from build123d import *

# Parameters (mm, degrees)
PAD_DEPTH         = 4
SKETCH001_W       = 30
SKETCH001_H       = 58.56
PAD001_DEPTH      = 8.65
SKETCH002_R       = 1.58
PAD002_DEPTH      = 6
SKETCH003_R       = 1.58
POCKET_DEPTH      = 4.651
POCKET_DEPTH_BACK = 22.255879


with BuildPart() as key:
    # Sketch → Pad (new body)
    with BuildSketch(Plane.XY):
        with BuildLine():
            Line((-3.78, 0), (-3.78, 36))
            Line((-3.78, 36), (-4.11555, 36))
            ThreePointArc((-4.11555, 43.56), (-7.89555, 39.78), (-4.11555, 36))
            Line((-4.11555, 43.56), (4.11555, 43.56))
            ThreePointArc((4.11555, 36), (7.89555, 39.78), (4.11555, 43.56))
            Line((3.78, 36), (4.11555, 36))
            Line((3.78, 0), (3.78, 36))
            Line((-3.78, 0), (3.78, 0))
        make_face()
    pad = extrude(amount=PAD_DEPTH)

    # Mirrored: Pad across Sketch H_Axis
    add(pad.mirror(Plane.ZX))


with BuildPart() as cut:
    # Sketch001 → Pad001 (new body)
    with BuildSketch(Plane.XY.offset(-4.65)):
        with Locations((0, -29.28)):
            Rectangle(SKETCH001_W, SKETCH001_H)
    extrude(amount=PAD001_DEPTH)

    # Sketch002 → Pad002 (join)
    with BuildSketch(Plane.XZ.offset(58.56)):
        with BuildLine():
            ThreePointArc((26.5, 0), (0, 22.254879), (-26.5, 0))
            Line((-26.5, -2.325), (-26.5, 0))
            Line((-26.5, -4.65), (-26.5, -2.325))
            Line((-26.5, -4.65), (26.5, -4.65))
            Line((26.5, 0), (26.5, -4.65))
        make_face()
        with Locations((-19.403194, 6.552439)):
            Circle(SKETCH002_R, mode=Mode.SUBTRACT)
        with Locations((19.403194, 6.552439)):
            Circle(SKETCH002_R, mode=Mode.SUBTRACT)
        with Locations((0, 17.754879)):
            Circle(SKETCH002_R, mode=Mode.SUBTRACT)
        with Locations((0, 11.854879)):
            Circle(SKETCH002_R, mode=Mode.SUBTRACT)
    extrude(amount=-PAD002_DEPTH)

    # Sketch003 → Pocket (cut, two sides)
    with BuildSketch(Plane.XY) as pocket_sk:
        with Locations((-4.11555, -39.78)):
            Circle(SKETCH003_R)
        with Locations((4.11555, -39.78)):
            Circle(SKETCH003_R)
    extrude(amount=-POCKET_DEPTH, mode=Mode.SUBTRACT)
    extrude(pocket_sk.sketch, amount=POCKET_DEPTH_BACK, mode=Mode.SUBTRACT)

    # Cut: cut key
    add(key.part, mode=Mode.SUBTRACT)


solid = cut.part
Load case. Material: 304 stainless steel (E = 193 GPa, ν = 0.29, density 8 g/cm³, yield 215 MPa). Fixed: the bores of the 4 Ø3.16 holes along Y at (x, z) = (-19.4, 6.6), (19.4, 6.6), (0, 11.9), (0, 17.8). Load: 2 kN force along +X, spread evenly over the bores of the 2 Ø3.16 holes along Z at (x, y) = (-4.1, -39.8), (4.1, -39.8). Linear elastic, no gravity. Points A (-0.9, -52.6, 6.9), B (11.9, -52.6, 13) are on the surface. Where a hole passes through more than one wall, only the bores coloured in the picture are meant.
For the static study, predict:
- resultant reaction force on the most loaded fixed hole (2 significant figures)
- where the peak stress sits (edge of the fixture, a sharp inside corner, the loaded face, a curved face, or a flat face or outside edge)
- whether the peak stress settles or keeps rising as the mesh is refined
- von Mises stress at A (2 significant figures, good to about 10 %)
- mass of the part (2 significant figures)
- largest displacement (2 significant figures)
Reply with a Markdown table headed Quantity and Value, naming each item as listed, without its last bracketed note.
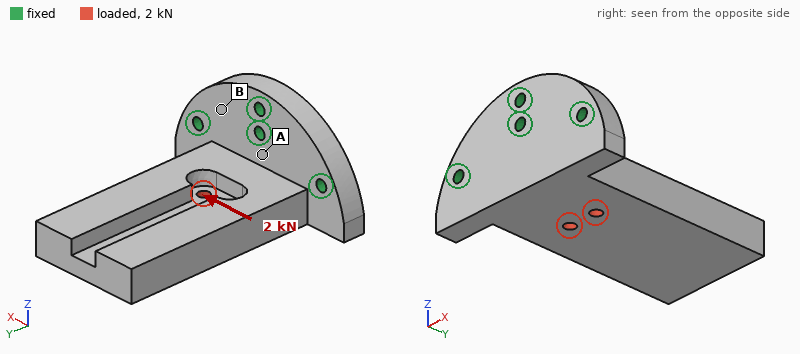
| Quantity | Value |
|---|---|
| resultant reaction force on the most loaded fixed hole | 1.3 kN |
| where the peak stress sits | edge of the fixture |
| whether the peak stress settles or keeps rising as the mesh is refined | keeps rising |
| von Mises stress at A | 21 MPa |
| mass of the part | 150 g |
| largest displacement | 16 µm |
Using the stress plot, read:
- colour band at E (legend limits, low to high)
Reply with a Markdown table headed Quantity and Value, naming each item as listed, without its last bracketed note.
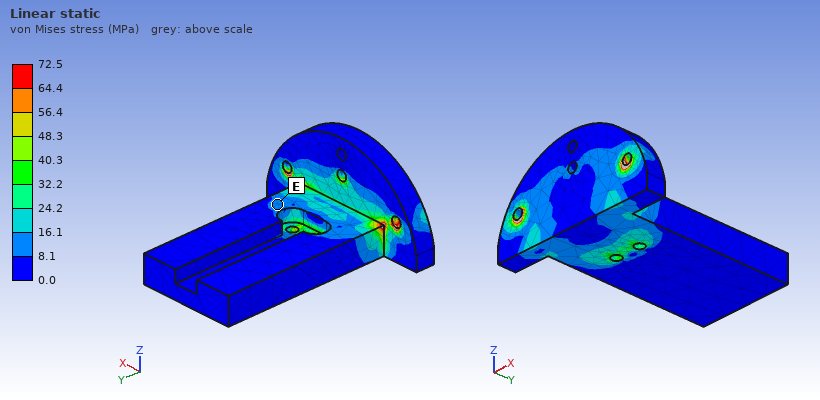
| Quantity | Value |
|---|---|
| colour band at E | 8.1 to 16.1 MPa |
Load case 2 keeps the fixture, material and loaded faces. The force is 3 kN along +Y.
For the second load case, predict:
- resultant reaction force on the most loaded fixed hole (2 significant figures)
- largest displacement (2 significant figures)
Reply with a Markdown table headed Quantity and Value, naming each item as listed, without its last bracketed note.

| Quantity | Value |
|---|---|
| resultant reaction force on the most loaded fixed hole | 1.3 kN |
| largest displacement | 82 µm |
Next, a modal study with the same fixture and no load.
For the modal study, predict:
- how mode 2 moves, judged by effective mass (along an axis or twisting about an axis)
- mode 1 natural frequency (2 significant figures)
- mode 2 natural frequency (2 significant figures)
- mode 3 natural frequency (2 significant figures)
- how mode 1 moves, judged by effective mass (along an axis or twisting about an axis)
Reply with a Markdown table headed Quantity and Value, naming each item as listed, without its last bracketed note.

| Quantity | Value |
|---|---|
| how mode 2 moves, judged by effective mass | along X |
| mode 1 natural frequency | 1600 Hz |
| mode 2 natural frequency | 4200 Hz |
| mode 3 natural frequency | 6400 Hz |
| how mode 1 moves, judged by effective mass | along Z |
